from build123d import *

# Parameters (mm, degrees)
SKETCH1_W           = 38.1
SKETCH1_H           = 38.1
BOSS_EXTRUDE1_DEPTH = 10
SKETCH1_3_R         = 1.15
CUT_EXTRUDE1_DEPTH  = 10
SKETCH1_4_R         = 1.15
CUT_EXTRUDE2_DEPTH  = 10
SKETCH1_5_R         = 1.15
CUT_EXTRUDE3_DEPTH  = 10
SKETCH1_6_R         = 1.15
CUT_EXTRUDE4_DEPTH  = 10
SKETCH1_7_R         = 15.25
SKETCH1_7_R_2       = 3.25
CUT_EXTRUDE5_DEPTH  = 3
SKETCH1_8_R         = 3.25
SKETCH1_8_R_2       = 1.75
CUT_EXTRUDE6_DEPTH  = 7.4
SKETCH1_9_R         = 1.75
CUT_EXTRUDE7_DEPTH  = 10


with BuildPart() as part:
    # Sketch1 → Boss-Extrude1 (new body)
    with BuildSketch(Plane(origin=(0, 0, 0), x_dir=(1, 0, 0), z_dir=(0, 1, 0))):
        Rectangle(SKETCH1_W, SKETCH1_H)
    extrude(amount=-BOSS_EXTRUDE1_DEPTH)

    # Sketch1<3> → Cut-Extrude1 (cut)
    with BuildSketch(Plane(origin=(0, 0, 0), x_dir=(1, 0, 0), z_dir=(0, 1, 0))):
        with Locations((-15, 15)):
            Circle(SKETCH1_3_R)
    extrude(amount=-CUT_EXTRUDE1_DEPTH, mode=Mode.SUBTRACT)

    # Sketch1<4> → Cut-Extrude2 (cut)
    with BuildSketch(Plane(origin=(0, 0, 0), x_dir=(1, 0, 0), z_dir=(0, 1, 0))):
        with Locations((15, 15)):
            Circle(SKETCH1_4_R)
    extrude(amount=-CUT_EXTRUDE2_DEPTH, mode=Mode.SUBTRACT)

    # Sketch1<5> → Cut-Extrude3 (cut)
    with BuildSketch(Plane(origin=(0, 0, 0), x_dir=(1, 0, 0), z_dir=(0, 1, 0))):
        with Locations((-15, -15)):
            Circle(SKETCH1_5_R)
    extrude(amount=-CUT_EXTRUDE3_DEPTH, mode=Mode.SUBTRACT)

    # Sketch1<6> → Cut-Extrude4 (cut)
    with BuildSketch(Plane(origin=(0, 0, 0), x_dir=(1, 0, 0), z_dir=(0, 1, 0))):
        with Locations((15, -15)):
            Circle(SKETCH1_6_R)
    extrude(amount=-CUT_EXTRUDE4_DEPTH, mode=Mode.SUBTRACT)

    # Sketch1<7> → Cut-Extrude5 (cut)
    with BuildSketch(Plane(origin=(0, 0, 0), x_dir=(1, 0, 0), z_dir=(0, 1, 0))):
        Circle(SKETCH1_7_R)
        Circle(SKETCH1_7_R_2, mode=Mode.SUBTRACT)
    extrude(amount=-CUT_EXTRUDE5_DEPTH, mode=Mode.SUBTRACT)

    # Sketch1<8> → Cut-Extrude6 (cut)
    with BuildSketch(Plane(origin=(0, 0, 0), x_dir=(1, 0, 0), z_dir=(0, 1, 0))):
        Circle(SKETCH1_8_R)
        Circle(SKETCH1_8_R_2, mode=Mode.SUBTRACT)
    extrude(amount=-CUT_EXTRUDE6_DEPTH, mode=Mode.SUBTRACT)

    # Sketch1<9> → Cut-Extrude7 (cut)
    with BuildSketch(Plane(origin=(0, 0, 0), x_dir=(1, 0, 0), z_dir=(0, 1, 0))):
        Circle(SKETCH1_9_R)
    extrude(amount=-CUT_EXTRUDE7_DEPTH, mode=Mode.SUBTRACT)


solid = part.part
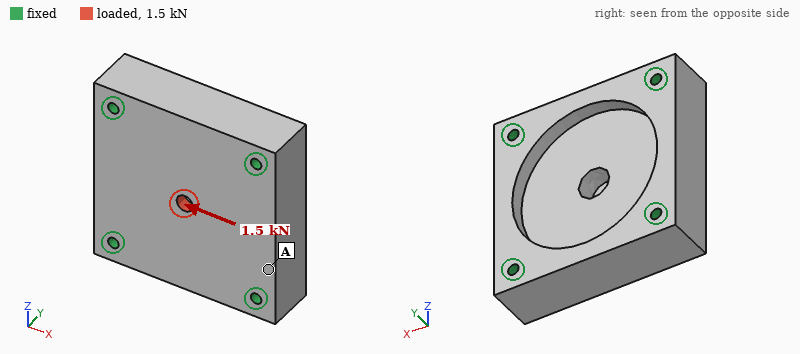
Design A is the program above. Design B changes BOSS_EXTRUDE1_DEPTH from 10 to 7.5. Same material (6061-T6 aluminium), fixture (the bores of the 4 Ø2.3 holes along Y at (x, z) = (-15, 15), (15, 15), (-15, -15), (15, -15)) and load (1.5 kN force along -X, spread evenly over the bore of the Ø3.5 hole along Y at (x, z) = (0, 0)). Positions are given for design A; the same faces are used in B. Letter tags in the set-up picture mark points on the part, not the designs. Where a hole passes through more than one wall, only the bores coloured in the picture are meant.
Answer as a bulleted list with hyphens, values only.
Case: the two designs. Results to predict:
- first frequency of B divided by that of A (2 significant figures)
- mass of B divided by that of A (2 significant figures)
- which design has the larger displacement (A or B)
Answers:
- 0.85
- 0.70
- B
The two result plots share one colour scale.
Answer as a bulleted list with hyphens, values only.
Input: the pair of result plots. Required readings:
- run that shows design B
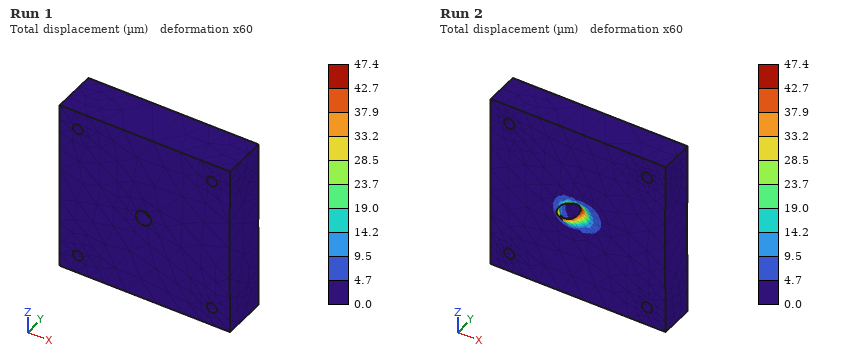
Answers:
- Run 2
